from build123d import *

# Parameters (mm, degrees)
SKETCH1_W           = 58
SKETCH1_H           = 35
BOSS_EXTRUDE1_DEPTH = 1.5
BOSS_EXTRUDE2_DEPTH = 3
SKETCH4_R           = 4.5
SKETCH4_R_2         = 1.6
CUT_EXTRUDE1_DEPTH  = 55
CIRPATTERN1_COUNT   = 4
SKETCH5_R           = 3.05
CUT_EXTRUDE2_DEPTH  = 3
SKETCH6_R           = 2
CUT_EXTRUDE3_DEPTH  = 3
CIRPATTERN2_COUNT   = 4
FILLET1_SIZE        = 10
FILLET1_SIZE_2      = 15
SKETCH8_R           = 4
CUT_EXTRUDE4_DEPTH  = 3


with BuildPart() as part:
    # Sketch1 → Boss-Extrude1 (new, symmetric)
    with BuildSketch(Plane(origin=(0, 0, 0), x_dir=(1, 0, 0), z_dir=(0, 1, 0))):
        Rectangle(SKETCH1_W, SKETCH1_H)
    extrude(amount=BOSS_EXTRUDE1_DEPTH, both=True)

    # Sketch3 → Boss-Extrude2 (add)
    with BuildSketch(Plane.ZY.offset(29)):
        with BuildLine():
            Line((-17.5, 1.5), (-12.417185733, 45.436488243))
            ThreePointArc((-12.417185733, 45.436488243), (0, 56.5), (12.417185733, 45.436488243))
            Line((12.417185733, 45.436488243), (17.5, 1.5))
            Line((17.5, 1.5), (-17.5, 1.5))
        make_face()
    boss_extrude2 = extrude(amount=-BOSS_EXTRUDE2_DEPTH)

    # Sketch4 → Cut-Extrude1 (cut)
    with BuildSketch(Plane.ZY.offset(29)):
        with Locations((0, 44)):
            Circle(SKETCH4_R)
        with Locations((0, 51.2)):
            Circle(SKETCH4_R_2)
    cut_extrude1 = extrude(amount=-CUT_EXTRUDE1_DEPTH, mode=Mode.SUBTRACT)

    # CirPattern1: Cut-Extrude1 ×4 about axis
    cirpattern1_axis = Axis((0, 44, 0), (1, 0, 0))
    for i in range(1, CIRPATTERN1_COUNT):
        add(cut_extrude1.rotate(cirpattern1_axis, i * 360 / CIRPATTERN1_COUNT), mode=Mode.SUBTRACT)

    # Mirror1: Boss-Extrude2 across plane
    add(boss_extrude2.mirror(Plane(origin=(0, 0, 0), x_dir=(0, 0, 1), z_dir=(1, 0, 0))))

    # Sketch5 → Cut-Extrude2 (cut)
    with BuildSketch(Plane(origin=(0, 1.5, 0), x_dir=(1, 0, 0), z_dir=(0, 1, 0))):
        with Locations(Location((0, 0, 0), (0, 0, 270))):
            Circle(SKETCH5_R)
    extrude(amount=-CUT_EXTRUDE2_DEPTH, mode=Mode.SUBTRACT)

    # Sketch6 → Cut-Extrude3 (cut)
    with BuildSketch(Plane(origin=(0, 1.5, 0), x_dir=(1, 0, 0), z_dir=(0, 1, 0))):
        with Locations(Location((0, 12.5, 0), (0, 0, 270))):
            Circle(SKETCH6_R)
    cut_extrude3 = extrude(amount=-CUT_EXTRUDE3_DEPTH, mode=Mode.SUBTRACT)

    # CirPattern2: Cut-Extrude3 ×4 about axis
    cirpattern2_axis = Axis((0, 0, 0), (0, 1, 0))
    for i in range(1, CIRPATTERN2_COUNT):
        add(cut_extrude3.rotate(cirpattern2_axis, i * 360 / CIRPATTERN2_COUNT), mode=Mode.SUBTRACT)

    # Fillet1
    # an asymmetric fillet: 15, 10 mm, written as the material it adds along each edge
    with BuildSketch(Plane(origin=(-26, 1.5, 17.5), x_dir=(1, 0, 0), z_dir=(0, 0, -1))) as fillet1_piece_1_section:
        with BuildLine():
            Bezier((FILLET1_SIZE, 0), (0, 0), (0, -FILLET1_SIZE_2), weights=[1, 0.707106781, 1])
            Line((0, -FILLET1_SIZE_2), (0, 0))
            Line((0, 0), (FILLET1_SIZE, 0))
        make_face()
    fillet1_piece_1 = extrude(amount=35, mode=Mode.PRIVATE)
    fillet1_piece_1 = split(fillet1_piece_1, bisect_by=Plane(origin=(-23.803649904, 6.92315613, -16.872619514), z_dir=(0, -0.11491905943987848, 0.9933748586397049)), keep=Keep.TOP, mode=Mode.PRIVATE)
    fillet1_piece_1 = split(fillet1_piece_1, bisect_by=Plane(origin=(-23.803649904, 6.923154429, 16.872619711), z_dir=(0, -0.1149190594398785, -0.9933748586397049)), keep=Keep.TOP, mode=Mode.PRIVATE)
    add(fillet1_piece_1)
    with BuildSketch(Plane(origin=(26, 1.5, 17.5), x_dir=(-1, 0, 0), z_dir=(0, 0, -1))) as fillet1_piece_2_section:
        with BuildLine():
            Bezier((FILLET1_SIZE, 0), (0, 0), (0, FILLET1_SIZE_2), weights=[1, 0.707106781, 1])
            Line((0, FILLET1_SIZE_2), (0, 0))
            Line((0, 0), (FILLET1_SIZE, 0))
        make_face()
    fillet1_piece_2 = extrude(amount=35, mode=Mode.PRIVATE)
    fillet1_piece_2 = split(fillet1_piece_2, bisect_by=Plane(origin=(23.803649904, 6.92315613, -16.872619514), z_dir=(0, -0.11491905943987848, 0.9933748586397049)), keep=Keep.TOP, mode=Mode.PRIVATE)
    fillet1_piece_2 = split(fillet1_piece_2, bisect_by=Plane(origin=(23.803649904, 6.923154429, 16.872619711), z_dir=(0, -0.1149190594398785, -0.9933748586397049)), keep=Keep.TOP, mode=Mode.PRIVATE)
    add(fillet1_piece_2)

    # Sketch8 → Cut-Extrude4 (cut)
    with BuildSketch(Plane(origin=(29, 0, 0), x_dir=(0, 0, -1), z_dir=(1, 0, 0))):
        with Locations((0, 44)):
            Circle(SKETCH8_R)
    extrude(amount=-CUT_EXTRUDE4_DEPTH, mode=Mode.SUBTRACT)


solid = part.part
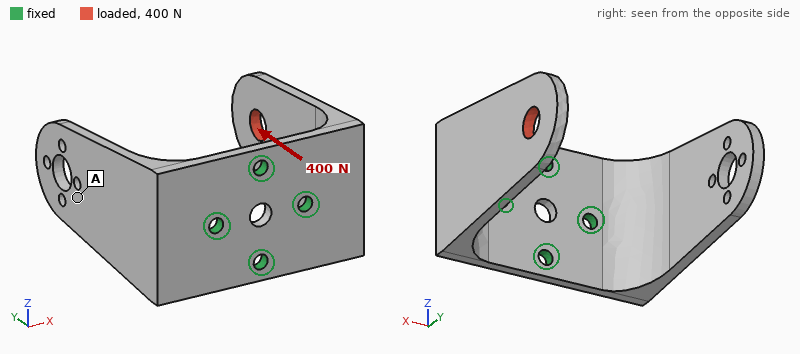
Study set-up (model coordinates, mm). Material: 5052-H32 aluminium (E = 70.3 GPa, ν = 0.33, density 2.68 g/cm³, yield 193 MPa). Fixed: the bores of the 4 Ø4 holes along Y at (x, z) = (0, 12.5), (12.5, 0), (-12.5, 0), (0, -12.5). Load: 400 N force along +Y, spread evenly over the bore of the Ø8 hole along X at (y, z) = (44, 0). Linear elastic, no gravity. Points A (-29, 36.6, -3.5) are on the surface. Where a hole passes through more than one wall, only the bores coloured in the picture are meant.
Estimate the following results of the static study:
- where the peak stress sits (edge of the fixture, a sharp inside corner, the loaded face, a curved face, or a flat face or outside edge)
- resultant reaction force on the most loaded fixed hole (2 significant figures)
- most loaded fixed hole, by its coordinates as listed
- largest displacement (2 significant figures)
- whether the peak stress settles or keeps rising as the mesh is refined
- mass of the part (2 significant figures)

edge of the fixture
590 N
(12.5, 0)
0.37 mm
keeps rising
45 g
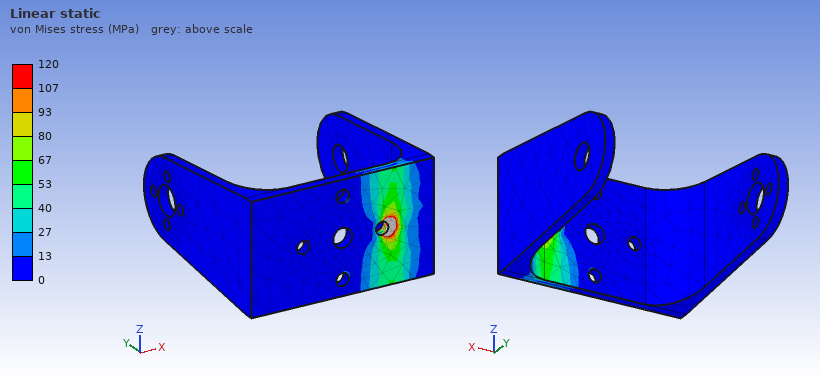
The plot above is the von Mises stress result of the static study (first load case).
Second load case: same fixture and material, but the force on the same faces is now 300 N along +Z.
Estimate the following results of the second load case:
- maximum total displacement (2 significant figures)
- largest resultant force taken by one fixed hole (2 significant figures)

0.52 mm
280 N
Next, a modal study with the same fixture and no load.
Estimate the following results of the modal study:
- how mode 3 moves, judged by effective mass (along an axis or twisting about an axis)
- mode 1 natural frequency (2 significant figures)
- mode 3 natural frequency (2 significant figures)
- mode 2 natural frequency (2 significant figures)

along Z
970 Hz
1800 Hz
1000 Hz
